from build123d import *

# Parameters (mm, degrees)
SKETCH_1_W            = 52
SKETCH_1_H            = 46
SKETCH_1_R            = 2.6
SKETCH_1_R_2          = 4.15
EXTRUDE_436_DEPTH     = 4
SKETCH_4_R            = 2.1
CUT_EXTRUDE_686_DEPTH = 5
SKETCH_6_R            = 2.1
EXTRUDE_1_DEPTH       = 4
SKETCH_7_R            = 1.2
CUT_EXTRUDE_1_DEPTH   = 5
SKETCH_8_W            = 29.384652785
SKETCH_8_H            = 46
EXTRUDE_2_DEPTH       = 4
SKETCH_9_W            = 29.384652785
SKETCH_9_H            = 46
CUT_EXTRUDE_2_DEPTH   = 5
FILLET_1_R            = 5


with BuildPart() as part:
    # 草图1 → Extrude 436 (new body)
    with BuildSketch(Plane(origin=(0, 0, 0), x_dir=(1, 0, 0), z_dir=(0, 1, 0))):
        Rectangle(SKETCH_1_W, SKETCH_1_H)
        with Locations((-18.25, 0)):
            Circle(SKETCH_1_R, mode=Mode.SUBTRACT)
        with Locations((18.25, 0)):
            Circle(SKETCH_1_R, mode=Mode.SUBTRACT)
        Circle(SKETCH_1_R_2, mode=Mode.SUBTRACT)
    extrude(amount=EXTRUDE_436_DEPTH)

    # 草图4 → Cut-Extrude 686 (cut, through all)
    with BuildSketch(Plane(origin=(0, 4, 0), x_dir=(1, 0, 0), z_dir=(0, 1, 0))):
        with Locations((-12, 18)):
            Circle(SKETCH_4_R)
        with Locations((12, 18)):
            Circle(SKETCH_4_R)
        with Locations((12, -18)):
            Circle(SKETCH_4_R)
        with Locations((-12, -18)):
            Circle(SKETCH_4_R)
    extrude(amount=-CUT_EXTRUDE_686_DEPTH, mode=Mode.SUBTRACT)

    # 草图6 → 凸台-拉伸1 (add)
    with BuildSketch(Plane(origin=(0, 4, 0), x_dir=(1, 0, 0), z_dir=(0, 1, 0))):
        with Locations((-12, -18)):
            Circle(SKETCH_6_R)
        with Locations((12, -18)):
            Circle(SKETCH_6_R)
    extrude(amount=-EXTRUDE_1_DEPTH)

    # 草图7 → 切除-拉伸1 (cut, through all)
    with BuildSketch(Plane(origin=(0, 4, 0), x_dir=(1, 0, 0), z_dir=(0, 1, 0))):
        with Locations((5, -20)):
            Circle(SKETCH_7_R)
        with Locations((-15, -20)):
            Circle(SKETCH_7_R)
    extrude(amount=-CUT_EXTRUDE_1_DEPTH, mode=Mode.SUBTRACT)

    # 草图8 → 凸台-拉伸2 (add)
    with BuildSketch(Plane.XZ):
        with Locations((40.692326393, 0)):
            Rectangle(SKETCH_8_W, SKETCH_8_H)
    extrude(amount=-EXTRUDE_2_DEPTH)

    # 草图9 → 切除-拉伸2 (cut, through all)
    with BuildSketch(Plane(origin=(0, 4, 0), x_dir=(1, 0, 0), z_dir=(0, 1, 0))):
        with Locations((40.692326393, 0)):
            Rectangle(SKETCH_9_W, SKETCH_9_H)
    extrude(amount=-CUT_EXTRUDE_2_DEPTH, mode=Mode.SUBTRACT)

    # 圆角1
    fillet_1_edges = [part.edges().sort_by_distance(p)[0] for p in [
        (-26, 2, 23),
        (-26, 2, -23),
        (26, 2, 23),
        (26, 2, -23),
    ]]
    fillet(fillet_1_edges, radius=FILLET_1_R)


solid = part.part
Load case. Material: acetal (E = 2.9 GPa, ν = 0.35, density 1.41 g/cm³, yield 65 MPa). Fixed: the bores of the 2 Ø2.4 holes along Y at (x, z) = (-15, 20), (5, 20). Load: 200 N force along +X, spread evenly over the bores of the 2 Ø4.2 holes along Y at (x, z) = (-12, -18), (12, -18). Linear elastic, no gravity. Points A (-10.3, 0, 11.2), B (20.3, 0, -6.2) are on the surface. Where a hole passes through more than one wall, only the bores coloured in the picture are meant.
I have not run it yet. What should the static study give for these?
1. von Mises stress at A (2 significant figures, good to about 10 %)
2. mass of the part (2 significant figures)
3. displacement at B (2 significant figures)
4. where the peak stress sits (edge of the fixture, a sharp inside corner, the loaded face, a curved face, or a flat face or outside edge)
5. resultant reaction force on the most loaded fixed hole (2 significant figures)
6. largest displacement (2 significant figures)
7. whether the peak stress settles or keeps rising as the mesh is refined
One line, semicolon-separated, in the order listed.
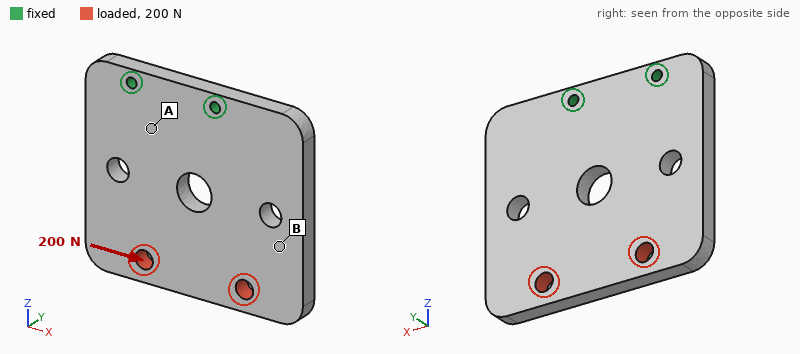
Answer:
6.0 MPa; 13 g; 0.20 mm; edge of the fixture; 370 N; 0.28 mm; keeps rising
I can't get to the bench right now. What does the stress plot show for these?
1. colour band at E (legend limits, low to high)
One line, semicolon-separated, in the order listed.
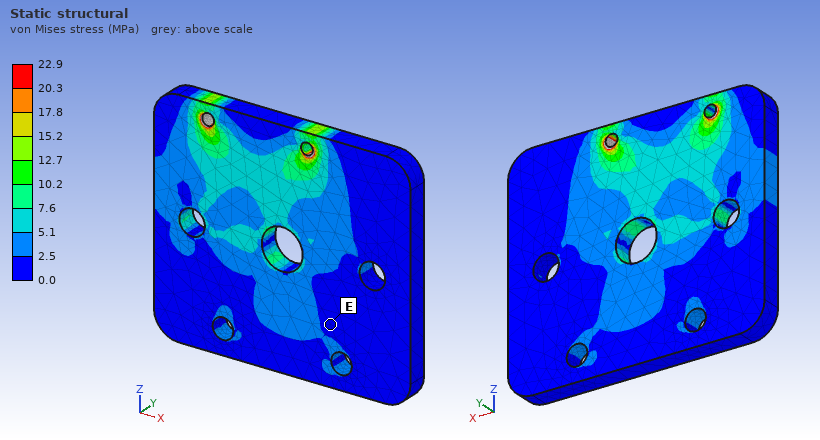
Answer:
0.0 to 2.5 MPa
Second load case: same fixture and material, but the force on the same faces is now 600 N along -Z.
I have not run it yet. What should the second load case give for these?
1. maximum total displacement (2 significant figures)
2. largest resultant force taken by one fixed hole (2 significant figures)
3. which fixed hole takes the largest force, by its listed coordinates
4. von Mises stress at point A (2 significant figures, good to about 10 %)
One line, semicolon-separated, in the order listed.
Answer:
0.15 mm; 440 N; (5, 20); 3.4 MPa
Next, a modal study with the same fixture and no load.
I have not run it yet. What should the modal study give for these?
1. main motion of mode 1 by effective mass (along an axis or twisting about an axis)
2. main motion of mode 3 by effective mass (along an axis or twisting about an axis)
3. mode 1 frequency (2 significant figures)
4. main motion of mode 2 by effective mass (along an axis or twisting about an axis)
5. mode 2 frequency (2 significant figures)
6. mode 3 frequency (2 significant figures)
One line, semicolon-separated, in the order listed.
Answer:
along Y; along X; 420 Hz; twisting about Z; 820 Hz; 1900 Hz
